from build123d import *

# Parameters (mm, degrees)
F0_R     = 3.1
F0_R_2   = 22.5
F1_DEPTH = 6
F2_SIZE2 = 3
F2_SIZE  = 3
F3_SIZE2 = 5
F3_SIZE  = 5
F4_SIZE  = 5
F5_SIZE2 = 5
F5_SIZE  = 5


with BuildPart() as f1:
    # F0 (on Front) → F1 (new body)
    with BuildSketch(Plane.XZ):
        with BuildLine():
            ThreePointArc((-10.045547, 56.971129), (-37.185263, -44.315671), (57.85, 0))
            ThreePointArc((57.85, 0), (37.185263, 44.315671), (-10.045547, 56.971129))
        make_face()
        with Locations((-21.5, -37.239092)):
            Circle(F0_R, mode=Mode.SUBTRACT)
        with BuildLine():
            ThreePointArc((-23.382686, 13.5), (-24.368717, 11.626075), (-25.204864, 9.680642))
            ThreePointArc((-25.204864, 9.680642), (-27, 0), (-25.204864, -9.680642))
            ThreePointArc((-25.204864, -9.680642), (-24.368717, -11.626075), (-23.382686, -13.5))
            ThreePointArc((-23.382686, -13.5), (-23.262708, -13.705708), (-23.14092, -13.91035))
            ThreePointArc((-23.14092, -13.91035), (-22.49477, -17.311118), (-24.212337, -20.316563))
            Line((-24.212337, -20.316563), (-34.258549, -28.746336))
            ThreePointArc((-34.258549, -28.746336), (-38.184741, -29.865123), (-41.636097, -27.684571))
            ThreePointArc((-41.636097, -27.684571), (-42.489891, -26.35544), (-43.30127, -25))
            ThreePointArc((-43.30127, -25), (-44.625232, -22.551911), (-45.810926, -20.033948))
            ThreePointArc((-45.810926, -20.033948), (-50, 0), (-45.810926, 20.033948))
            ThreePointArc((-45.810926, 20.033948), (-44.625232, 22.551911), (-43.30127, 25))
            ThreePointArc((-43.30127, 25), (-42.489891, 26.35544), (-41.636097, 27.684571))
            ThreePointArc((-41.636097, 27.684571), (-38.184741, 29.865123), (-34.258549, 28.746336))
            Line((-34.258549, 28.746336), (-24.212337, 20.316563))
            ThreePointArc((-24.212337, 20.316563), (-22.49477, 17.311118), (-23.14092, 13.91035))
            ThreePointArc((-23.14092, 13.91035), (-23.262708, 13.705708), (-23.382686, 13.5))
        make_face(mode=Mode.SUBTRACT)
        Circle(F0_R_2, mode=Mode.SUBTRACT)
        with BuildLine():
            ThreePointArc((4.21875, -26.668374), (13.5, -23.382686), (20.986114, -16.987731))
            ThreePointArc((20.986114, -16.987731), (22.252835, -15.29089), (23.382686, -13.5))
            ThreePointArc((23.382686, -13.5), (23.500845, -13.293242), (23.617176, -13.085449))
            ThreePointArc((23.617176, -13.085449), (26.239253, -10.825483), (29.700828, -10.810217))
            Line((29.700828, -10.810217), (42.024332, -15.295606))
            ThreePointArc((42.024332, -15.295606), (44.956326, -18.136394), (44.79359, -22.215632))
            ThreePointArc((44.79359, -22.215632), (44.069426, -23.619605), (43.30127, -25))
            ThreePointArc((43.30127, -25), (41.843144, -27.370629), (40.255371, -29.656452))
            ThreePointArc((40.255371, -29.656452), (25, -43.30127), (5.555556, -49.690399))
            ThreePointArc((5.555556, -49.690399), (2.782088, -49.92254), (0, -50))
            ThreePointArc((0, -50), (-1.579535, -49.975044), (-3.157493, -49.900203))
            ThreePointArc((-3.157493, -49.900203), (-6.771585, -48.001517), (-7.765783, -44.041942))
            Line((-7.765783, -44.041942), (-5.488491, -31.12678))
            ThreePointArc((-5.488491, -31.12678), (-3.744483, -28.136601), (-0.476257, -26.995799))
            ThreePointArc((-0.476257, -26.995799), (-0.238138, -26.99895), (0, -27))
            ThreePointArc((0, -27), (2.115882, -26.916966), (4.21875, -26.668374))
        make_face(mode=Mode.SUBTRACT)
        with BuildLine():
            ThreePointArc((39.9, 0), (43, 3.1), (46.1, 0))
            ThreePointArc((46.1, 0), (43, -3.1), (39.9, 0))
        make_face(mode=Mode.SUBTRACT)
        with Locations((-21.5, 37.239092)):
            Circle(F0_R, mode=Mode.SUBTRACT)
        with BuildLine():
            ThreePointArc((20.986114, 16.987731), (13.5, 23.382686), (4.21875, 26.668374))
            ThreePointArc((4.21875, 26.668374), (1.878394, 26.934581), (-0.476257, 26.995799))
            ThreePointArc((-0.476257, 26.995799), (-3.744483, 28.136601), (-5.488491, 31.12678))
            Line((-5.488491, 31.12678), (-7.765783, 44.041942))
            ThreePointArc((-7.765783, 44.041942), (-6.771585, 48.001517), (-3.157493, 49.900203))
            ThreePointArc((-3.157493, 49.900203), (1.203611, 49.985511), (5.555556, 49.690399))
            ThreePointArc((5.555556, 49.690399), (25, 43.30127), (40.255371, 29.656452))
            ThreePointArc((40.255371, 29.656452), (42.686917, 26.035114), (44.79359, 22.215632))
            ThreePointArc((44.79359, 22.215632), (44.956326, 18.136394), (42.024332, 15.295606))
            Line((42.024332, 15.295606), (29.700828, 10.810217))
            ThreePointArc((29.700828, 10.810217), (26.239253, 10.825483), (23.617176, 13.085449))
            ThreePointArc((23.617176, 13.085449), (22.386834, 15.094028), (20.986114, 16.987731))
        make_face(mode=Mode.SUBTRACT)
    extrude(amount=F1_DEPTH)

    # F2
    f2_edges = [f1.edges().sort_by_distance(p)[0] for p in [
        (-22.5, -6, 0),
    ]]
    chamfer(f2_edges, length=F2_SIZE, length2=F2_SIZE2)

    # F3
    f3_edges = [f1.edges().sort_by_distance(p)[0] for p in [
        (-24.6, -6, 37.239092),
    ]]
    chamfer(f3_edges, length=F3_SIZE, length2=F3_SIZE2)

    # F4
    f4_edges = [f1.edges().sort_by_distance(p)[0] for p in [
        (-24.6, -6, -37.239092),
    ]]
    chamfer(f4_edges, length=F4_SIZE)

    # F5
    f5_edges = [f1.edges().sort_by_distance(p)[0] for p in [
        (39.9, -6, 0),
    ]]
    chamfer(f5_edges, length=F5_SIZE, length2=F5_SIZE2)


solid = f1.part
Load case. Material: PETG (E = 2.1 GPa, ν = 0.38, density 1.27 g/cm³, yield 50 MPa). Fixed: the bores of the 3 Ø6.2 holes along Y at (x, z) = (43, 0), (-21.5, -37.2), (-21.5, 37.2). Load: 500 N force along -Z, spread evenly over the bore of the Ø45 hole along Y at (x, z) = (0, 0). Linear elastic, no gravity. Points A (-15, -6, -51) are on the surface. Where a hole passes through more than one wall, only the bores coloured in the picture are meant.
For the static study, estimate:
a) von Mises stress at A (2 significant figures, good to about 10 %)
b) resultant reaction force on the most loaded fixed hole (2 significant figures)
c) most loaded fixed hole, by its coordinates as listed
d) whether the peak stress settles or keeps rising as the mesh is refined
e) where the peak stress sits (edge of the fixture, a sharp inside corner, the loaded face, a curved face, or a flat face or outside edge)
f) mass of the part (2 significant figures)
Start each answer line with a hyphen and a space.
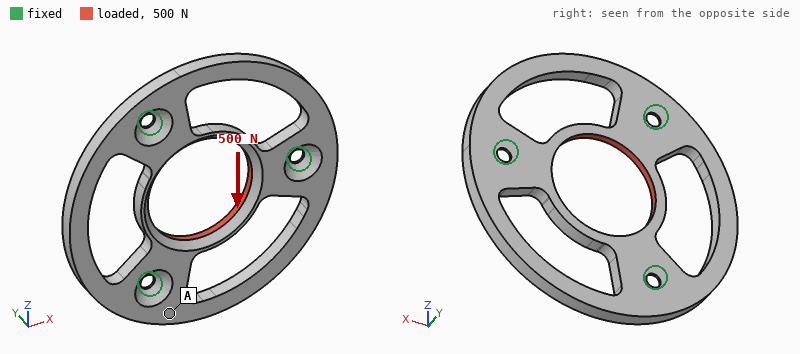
- 1.8 MPa
- 250 N
- (43, 0)
- keeps rising
- edge of the fixture
- 37 g
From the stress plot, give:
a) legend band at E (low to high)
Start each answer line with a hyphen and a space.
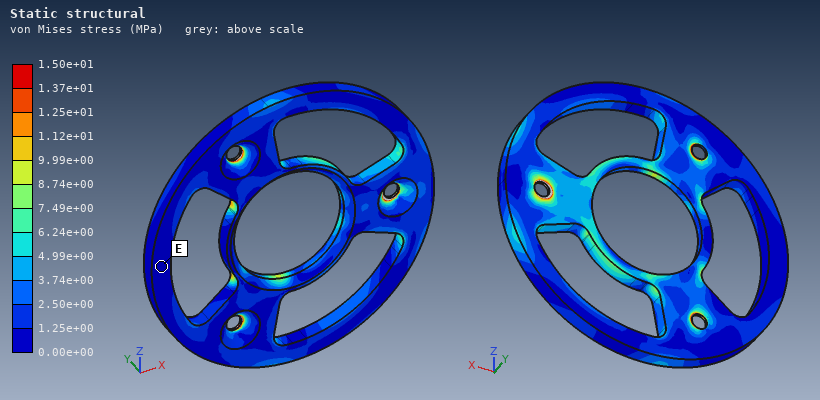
- 0.00e+00 to 1.25e+00 MPa
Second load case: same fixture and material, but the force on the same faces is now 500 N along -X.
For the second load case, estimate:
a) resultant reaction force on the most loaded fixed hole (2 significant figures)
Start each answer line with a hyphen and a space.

- 220 N
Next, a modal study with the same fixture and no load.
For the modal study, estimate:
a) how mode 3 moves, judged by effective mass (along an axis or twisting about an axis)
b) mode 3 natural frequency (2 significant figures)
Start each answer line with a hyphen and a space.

- along Y
- 690 Hz
